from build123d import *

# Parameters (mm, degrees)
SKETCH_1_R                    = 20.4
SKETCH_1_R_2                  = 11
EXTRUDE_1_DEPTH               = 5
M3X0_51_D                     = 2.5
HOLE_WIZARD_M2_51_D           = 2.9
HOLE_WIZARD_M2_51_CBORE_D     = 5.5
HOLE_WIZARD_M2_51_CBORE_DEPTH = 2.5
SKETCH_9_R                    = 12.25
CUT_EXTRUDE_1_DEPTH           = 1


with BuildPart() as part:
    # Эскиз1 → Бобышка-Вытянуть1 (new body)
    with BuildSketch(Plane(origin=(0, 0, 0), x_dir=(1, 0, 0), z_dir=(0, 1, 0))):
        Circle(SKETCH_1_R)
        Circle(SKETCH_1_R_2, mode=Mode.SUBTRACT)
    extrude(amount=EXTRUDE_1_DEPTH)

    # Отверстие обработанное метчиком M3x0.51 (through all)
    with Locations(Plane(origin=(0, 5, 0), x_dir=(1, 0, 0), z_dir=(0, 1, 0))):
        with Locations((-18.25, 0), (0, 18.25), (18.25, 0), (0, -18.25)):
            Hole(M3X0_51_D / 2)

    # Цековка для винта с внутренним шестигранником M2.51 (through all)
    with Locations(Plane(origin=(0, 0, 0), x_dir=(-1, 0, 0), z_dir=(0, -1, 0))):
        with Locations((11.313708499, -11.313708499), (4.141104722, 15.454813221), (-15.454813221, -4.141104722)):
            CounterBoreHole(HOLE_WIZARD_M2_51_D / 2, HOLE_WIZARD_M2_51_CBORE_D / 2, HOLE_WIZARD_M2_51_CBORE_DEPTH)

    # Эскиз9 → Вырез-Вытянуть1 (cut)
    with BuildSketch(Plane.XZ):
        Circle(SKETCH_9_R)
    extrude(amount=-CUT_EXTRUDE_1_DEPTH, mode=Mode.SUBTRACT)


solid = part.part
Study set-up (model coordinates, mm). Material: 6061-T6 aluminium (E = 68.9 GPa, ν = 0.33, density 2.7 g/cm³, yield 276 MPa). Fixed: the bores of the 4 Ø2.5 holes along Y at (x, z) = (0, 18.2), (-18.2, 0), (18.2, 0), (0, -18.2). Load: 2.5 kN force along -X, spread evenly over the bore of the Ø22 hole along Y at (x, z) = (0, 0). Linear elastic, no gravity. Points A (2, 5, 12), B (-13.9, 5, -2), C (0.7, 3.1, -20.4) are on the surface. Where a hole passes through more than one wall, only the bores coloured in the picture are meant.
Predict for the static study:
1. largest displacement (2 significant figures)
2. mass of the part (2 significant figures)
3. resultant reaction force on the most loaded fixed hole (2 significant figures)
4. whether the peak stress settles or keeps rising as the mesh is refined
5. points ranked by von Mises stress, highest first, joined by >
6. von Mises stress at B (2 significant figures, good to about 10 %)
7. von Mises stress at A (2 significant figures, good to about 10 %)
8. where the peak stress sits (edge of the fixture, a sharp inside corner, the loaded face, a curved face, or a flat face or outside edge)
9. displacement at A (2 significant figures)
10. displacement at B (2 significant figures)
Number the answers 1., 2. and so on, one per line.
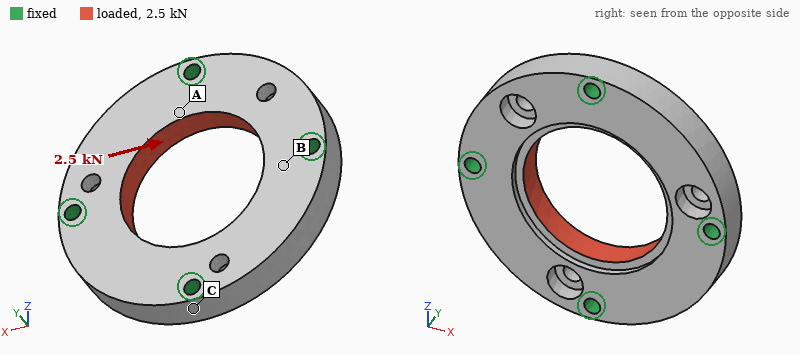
1. 4.4 µm
2. 11 g
3. 690 N
4. keeps rising
5. B > A > C
6. 21 MPa
7. 11 MPa
8. edge of the fixture
9. 3.3 µm
10. 1.5 µm
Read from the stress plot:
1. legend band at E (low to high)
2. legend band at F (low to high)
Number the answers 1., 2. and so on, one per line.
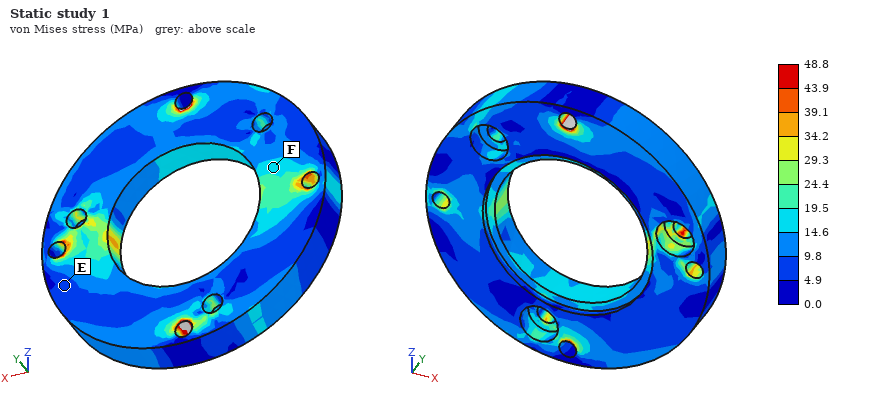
1. 4.9 to 9.8 MPa
2. 14.6 to 19.5 MPa
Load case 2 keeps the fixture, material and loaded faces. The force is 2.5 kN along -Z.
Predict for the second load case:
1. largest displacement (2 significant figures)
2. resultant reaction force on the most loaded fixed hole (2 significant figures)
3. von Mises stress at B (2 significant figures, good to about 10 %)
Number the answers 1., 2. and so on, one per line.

1. 4.4 µm
2. 690 N
3. 10 MPa
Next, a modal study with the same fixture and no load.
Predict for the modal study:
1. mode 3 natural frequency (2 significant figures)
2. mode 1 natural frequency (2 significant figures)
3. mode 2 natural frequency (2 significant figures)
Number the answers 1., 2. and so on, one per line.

1. 28 kHz
2. 25 kHz
3. 26 kHz
